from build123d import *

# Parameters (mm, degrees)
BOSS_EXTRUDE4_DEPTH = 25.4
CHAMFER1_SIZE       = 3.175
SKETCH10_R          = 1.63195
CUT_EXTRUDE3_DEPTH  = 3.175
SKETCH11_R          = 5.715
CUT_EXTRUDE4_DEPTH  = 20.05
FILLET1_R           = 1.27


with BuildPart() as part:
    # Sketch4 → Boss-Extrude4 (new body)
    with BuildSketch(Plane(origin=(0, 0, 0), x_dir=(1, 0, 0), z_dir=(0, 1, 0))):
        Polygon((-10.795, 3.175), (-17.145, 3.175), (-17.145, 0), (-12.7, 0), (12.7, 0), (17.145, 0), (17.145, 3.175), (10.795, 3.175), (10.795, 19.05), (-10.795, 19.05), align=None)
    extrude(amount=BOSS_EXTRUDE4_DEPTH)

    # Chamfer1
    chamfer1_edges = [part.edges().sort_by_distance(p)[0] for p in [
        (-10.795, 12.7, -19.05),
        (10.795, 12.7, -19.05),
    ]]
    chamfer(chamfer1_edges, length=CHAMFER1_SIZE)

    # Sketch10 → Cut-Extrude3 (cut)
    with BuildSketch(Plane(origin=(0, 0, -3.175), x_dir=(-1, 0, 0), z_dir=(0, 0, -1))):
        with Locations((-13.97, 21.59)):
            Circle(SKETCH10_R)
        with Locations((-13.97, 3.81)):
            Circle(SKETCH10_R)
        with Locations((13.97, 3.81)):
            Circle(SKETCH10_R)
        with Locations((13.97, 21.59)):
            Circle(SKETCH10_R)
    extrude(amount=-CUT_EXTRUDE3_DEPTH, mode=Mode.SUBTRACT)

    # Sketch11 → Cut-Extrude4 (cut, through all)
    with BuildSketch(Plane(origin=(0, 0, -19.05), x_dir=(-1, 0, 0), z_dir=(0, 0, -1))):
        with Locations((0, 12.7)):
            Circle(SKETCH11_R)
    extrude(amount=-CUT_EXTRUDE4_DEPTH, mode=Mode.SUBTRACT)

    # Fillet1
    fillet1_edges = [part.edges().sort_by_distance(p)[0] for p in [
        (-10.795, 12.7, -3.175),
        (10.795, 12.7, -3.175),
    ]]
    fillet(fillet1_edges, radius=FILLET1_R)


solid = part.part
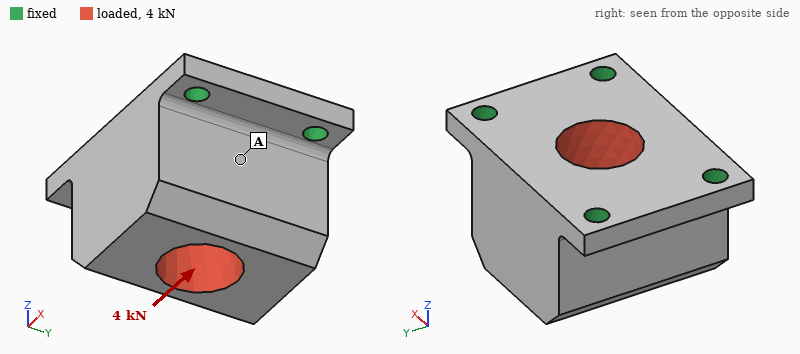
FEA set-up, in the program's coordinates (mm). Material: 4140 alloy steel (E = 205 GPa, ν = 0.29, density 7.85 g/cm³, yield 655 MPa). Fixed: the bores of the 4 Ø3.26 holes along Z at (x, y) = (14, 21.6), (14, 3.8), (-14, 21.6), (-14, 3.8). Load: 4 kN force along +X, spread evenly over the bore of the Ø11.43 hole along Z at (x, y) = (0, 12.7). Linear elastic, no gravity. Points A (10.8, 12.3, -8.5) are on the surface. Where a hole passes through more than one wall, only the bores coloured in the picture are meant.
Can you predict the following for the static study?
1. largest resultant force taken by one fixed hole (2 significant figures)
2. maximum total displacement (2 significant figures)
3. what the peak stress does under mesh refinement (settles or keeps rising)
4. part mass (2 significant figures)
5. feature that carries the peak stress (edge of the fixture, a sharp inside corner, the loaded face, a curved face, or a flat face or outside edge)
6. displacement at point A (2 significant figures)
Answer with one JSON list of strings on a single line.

["1.2 kN", "4.8 µm", "keeps rising", "72 g", "edge of the fixture", "2.8 µm"]
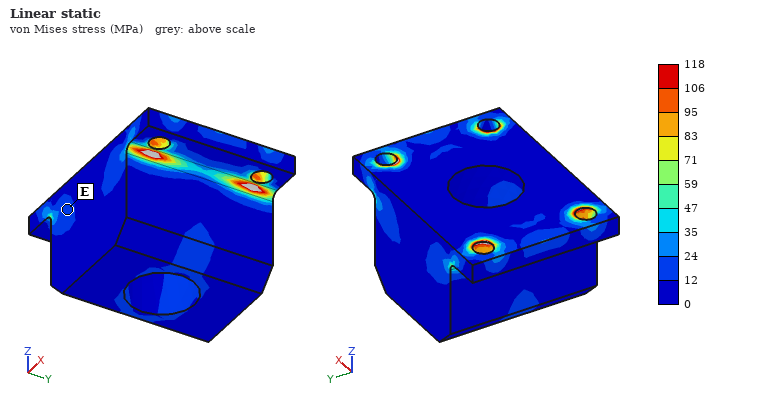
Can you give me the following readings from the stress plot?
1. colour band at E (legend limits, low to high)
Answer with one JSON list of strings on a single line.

["12 to 24 MPa"]
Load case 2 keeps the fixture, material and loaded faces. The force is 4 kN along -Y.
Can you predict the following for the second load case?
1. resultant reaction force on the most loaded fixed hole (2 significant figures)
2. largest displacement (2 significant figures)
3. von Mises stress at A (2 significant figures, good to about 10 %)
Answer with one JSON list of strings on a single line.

["1.5 kN", "9.3 µm", "20 MPa"]
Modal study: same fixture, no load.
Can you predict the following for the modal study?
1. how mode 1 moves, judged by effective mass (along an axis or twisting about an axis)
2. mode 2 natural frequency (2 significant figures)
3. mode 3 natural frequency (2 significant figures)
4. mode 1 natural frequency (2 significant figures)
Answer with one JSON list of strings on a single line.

["along Y", "22 kHz", "22 kHz", "15 kHz"]
